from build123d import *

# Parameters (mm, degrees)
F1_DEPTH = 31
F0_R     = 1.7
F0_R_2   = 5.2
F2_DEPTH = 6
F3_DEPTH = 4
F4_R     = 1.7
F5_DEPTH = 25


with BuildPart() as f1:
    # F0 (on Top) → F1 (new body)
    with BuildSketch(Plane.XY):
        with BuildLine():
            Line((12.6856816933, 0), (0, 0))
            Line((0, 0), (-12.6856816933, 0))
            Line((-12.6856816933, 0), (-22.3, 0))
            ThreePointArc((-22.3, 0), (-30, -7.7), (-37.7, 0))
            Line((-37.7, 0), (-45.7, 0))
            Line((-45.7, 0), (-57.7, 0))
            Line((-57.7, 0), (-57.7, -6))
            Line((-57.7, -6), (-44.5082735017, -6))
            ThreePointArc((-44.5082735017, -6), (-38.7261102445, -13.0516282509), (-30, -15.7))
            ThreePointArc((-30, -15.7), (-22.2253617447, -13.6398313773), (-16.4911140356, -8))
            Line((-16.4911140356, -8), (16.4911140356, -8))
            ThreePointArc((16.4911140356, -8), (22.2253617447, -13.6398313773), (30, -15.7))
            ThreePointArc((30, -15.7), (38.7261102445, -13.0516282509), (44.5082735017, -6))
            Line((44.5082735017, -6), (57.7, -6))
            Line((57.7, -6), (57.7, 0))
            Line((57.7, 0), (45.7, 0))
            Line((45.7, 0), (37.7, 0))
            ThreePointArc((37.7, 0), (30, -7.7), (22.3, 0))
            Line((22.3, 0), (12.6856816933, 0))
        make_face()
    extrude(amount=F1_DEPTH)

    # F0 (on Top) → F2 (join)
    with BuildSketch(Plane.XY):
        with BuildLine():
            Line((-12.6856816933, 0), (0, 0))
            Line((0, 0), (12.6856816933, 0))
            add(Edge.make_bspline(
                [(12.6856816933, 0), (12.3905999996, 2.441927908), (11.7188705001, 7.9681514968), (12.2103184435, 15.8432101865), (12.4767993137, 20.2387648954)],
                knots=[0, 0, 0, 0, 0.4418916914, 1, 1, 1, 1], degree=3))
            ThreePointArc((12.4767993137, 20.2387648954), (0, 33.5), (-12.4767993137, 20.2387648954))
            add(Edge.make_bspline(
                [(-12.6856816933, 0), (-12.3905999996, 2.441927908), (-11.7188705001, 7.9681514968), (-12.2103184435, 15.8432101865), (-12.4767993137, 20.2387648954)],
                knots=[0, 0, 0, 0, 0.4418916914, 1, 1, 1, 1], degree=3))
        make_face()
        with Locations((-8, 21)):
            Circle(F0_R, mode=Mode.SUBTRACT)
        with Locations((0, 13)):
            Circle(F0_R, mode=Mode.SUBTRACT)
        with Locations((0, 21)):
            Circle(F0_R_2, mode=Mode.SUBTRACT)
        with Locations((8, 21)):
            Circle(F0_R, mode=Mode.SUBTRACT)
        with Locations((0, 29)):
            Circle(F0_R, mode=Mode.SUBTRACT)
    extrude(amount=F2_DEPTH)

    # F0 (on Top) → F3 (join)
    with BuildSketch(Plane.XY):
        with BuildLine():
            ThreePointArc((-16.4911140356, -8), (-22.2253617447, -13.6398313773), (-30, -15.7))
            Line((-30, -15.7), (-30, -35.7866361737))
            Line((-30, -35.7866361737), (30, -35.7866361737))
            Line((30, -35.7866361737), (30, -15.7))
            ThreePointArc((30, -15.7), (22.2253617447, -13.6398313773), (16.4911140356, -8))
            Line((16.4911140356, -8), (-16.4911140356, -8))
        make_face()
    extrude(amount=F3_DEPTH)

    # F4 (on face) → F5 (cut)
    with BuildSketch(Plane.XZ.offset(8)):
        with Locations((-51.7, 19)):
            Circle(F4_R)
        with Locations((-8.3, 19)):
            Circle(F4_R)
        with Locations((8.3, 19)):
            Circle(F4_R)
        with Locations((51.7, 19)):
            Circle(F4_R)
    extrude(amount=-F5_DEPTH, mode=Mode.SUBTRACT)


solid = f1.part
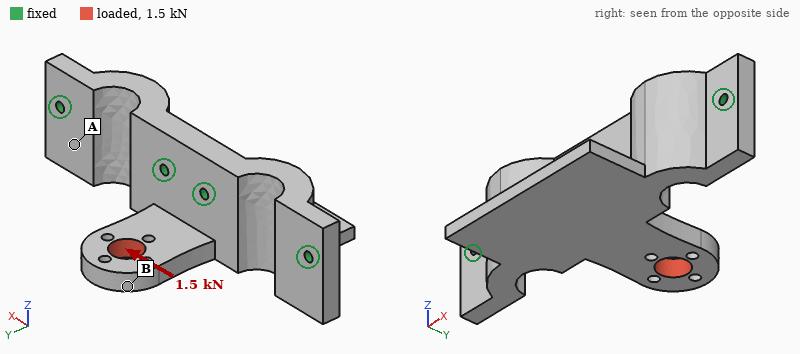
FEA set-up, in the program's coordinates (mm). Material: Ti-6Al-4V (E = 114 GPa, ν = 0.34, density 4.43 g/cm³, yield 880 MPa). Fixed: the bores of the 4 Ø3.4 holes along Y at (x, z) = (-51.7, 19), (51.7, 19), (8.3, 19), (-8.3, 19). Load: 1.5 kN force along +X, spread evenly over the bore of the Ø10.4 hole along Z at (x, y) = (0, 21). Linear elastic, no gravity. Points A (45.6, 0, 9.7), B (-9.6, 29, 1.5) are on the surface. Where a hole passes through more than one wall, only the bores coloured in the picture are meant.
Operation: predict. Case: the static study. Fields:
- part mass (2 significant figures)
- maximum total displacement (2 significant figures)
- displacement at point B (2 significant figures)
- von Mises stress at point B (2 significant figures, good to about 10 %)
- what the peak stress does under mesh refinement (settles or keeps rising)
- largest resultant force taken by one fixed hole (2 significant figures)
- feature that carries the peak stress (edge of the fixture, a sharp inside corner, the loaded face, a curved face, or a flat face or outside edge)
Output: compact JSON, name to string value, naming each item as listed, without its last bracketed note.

{"part mass": "180 g", "maximum total displacement": "55 µm", "displacement at point B": "51 µm", "von Mises stress at point B": "17 MPa", "what the peak stress does under mesh refinement": "keeps rising", "largest resultant force taken by one fixed hole": "1.5 kN", "feature that carries the peak stress": "edge of the fixture"}
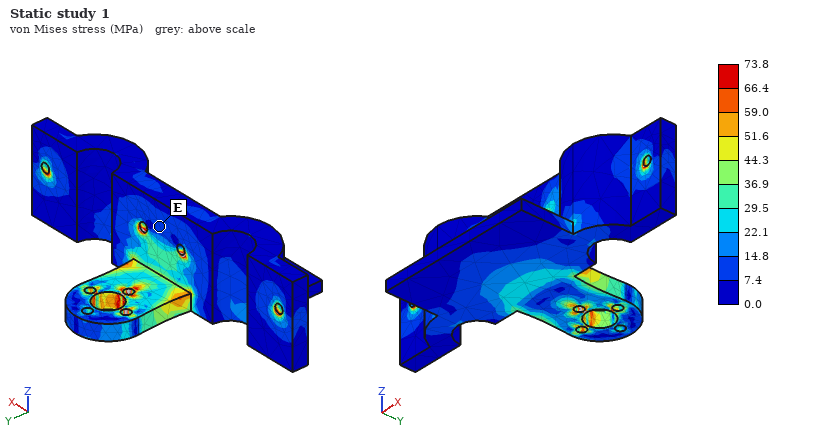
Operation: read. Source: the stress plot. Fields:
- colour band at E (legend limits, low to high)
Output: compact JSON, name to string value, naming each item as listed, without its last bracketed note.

{"colour band at E": "7.4 to 14.8 MPa"}
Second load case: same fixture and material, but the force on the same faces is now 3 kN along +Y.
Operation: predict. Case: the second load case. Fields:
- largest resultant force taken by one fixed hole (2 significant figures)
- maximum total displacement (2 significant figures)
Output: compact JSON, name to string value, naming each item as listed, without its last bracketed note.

{"largest resultant force taken by one fixed hole": "1.3 kN", "maximum total displacement": "72 µm"}
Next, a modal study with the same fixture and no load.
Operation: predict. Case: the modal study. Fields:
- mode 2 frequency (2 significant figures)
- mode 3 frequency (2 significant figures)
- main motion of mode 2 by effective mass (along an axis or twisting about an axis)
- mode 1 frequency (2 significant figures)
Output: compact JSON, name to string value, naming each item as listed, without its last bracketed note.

{"mode 2 frequency": "4700 Hz", "mode 3 frequency": "5800 Hz", "main motion of mode 2 by effective mass": "along Z", "mode 1 frequency": "3500 Hz"}
